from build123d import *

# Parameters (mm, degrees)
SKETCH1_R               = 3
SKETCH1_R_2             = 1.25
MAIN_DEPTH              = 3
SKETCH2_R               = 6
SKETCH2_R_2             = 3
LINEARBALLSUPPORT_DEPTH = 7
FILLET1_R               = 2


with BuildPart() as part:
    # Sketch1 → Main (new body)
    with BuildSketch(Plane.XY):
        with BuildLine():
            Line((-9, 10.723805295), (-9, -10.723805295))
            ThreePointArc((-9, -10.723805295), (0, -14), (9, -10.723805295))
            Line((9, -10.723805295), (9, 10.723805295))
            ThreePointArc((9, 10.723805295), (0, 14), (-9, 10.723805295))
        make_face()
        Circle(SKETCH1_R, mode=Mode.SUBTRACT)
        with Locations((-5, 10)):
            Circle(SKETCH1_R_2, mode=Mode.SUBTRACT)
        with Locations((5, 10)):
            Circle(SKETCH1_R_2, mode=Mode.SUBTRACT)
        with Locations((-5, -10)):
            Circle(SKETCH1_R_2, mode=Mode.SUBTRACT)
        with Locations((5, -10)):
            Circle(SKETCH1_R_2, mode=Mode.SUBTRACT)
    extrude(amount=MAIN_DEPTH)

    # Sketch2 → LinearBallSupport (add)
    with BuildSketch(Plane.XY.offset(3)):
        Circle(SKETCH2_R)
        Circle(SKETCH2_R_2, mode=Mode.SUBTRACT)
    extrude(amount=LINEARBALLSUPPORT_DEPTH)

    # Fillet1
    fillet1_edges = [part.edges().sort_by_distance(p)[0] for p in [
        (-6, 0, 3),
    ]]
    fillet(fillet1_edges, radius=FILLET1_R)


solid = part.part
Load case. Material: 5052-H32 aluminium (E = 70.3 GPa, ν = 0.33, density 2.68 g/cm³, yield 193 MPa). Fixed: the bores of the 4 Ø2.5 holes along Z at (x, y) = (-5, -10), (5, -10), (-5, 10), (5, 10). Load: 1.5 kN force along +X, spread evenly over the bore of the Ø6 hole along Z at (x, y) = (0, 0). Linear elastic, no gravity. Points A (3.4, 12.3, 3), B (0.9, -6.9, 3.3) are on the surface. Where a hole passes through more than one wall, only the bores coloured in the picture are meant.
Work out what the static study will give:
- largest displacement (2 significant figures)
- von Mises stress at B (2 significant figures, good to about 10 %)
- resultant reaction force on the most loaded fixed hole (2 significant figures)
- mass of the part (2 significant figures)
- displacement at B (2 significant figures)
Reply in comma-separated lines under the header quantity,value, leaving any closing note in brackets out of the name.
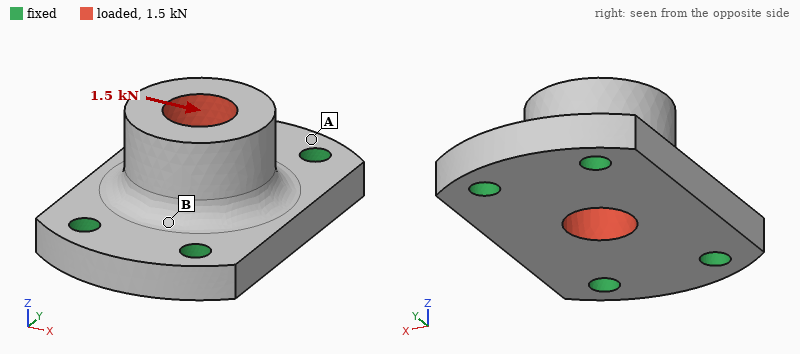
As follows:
quantity,value
largest displacement,17 µm
von Mises stress at B,71 MPa
resultant reaction force on the most loaded fixed hole,510 N
mass of the part,5.1 g
displacement at B,3.4 µm
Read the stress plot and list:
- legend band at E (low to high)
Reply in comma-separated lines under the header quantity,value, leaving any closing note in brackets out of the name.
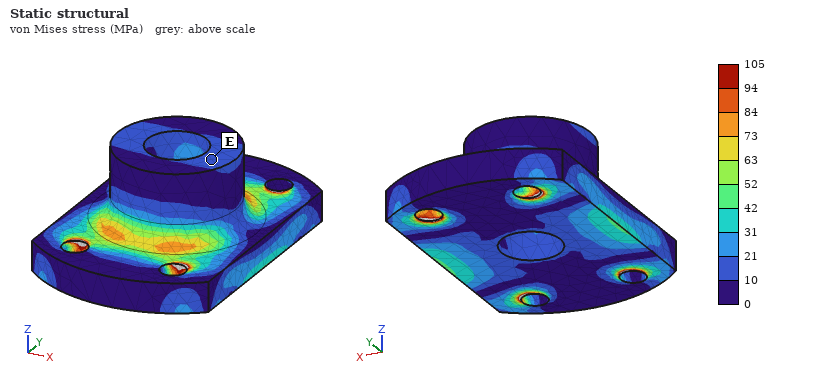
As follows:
quantity,value
legend band at E,10 to 21 MPa
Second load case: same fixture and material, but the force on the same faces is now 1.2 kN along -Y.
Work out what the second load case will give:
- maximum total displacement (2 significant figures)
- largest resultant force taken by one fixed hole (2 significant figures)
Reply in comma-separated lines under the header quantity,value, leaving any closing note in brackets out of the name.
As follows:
quantity,value
maximum total displacement,6.2 µm
largest resultant force taken by one fixed hole,330 N
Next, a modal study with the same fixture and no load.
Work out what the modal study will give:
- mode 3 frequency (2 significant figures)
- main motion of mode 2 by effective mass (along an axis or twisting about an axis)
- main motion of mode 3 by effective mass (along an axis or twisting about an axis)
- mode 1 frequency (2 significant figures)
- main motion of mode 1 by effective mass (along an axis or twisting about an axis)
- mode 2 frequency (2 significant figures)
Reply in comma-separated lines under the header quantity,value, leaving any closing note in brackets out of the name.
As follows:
quantity,value
mode 3 frequency,51 kHz
main motion of mode 2 by effective mass,along Z
main motion of mode 3 by effective mass,along Y
mode 1 frequency,30 kHz
main motion of mode 1 by effective mass,along X
mode 2 frequency,35 kHz
